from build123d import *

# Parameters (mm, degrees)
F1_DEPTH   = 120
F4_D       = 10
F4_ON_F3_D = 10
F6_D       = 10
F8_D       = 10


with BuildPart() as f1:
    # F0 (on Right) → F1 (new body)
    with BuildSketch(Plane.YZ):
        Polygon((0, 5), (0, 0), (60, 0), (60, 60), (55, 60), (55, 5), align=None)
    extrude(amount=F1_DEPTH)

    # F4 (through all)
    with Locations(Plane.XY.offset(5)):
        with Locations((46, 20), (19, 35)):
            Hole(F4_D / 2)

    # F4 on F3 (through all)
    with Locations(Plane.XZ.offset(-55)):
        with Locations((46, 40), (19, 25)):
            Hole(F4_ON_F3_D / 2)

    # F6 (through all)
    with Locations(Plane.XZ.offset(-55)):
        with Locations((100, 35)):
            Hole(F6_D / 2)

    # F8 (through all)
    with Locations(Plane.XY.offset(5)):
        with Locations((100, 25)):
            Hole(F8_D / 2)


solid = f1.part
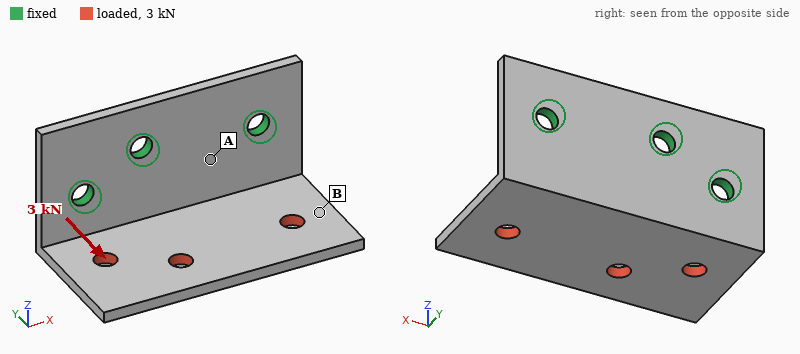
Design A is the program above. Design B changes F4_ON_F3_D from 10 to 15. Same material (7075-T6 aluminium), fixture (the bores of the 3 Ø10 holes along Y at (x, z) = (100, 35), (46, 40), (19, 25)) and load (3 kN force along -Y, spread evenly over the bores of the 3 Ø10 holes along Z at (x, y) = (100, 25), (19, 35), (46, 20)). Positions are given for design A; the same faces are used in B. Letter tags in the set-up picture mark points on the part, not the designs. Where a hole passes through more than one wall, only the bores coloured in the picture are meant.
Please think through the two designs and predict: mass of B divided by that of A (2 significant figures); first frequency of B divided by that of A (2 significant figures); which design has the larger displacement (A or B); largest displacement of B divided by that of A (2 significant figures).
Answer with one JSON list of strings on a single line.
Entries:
["0.99", "1.0", "A", "0.92"]
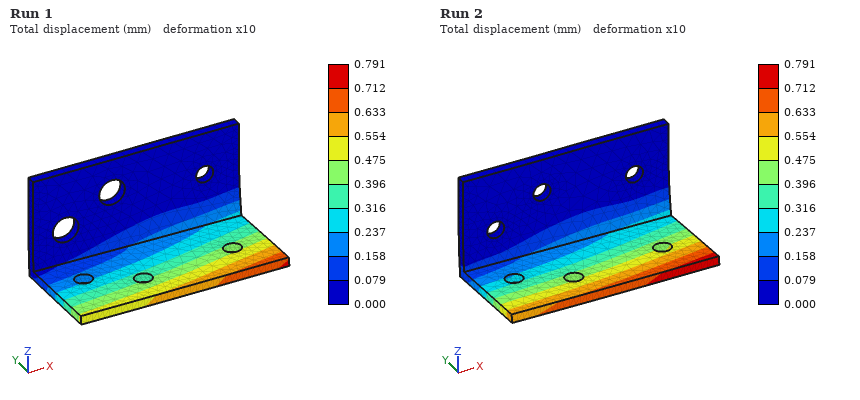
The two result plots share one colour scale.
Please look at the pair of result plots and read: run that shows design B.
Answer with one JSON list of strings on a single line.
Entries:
["Run 1"]
